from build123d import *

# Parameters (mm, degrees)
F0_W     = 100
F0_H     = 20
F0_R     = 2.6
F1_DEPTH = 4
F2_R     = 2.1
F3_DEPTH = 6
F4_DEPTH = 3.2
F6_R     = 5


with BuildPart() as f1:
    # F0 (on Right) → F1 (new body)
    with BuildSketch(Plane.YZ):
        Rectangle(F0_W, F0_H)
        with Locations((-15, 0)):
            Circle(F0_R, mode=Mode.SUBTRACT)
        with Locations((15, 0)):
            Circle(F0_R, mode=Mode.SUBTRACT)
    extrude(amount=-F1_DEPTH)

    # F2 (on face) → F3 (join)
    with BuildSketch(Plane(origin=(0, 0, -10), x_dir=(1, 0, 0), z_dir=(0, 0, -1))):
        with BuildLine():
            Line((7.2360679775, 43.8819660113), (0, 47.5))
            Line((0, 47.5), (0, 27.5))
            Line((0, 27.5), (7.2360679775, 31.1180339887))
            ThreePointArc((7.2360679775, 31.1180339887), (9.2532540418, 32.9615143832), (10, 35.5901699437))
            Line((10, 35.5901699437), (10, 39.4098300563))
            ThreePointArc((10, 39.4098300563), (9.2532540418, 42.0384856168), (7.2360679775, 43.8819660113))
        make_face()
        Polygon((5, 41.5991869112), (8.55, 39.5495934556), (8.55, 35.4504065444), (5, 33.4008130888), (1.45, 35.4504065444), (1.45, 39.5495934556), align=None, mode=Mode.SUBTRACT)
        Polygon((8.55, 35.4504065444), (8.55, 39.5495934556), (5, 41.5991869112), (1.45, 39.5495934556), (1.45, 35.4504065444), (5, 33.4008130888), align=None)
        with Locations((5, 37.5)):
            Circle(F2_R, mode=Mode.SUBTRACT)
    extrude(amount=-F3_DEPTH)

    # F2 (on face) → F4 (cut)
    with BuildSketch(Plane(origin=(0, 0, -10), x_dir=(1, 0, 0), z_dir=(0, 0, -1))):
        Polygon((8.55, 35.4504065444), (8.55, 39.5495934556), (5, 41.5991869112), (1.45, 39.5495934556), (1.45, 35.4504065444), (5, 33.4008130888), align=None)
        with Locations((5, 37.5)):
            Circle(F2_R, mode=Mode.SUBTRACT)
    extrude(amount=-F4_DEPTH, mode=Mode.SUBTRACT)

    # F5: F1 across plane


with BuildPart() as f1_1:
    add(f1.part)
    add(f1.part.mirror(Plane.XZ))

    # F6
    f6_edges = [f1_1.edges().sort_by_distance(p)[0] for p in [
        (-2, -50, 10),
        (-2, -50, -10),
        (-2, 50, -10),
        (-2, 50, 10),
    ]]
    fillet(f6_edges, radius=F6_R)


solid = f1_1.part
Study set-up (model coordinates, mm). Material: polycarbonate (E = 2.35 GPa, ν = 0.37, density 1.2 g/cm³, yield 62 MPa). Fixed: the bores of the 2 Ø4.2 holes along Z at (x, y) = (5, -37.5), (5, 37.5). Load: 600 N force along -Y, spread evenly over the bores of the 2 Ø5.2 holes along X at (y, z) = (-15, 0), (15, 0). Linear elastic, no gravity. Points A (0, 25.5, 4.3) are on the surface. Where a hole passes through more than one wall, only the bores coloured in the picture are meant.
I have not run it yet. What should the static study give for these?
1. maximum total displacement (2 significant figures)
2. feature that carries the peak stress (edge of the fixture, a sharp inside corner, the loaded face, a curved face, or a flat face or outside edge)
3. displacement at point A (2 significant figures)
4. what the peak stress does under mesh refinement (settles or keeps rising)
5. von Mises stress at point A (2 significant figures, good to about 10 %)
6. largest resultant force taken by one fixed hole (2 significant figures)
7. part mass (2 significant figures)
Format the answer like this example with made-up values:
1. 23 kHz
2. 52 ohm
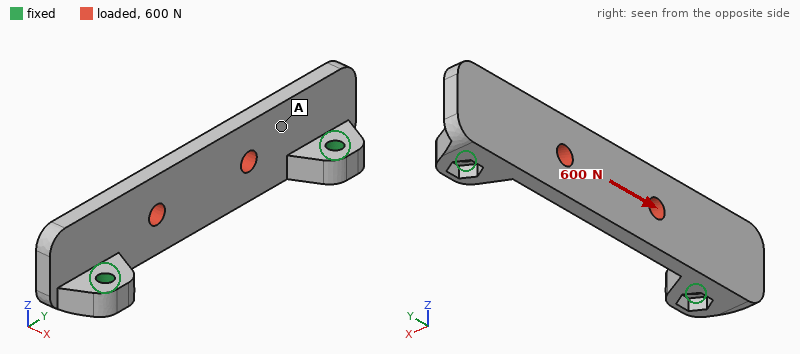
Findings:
1. 0.22 mm
2. edge of the fixture
3. 0.20 mm
4. keeps rising
5. 6.1 MPa
6. 300 N
7. 11 g
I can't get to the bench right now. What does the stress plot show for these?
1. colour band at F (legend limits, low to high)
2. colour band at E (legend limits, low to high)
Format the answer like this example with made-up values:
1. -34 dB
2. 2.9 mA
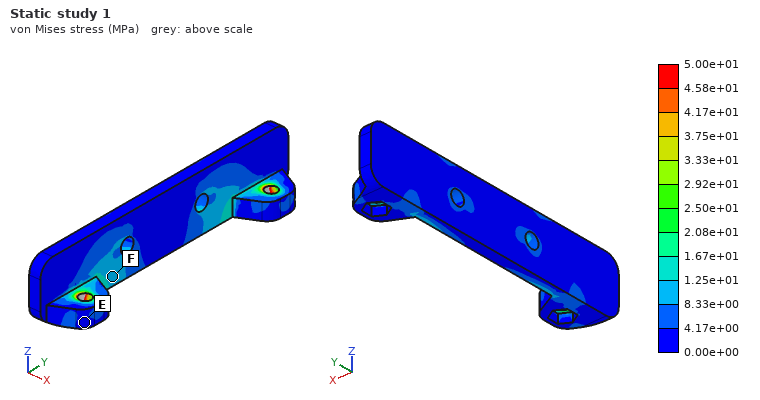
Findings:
1. 8.33e+00 to 1.25e+01 MPa
2. 0.00e+00 to 4.17e+00 MPa
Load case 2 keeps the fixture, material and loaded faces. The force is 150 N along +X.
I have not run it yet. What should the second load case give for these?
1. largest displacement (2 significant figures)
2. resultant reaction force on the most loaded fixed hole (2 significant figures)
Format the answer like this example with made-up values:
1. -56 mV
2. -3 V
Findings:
1. 1.00 mm
2. 120 N
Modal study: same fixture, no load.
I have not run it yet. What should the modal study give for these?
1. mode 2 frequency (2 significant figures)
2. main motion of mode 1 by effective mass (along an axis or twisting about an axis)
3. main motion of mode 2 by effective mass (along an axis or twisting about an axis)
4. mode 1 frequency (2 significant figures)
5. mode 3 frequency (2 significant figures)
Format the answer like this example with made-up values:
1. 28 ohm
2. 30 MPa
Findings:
1. 1700 Hz
2. along X
3. along Z
4. 1000 Hz
5. 1900 Hz
